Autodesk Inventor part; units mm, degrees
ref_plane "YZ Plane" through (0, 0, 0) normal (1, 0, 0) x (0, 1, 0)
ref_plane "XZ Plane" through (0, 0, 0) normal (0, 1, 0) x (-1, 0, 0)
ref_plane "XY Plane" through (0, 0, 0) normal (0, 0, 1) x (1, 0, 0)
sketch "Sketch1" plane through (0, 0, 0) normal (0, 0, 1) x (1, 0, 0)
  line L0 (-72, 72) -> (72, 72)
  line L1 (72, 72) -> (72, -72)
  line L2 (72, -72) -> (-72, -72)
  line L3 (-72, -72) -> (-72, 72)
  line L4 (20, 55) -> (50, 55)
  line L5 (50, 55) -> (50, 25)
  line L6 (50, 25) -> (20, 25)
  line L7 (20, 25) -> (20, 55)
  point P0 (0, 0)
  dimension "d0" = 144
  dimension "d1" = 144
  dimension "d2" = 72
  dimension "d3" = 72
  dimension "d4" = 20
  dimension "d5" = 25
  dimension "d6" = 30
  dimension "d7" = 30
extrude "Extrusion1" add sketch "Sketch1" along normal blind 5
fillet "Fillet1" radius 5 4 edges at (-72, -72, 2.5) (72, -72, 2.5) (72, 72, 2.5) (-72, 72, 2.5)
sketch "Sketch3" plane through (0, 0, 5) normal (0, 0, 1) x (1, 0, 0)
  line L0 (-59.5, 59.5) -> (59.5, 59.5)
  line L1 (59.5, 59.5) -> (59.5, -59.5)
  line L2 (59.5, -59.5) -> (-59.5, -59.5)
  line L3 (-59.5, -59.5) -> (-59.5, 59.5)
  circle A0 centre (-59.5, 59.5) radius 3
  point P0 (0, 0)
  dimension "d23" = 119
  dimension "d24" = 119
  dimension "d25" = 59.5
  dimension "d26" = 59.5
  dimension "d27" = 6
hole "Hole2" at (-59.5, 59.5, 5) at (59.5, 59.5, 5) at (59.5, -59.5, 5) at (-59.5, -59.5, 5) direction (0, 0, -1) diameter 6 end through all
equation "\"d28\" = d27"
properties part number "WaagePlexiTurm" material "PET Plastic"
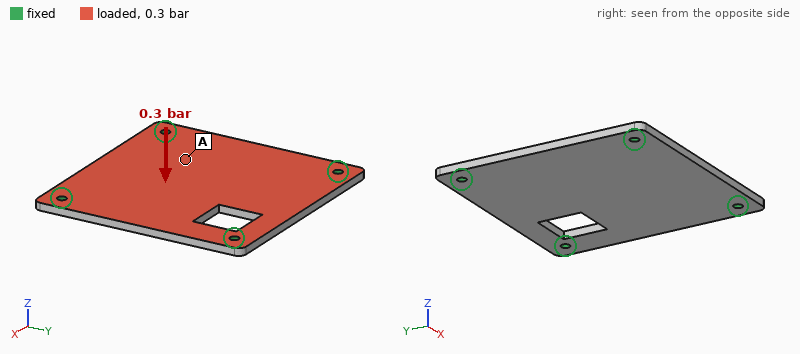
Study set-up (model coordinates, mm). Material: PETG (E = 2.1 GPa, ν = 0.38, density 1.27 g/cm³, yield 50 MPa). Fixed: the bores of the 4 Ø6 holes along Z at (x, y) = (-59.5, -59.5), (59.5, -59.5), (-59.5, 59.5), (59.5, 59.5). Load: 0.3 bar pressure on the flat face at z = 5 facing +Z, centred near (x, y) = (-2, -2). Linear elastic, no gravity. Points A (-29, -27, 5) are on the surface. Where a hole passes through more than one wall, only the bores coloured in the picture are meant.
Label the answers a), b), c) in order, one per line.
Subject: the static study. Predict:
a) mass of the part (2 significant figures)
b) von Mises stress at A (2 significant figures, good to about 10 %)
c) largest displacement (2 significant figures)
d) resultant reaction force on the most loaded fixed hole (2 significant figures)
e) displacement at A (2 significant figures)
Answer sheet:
a) 130 g
b) 3.5 MPa
c) 1.9 mm
d) 160 N
e) 1.3 mm
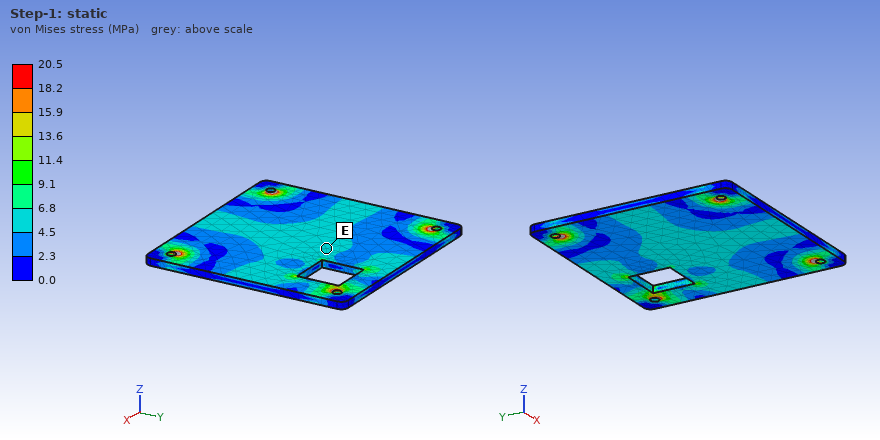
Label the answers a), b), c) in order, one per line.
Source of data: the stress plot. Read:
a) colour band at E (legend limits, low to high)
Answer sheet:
a) 4.5 to 6.8 MPa
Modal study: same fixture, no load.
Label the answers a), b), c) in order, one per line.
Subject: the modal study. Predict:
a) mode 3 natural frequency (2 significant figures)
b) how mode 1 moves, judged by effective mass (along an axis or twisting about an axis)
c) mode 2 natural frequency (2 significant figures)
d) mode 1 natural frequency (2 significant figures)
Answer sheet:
a) 510 Hz
b) along Z
c) 490 Hz
d) 300 Hz
